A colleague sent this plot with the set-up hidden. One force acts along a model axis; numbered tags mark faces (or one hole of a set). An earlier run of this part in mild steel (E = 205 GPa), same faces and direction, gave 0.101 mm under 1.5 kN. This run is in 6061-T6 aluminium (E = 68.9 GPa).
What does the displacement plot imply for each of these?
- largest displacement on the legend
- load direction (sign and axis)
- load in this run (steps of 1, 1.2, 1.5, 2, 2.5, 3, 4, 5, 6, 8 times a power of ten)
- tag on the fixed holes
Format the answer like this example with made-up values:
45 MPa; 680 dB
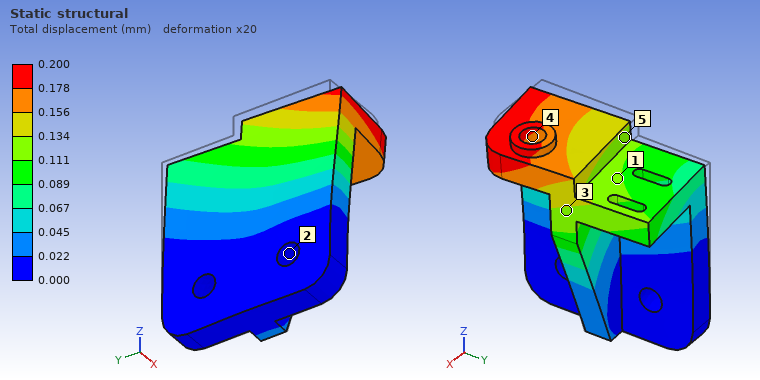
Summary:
0.200 mm; +X; 1 kN; 2
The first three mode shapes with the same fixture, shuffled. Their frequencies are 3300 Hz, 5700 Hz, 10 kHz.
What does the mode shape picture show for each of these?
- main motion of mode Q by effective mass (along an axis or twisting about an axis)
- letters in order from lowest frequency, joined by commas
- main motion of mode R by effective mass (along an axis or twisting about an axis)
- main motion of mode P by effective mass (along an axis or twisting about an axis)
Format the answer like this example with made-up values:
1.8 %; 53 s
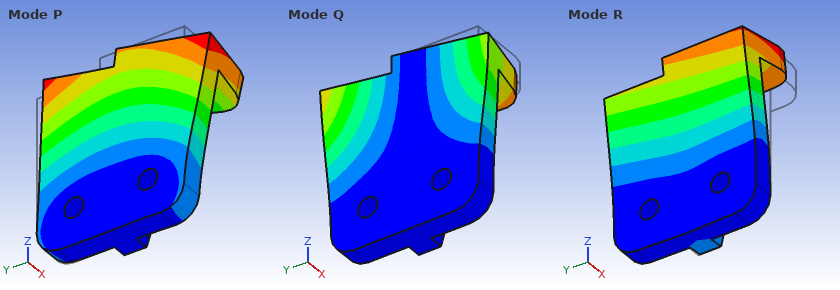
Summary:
along Y; R, Q, P; along X; along Y
